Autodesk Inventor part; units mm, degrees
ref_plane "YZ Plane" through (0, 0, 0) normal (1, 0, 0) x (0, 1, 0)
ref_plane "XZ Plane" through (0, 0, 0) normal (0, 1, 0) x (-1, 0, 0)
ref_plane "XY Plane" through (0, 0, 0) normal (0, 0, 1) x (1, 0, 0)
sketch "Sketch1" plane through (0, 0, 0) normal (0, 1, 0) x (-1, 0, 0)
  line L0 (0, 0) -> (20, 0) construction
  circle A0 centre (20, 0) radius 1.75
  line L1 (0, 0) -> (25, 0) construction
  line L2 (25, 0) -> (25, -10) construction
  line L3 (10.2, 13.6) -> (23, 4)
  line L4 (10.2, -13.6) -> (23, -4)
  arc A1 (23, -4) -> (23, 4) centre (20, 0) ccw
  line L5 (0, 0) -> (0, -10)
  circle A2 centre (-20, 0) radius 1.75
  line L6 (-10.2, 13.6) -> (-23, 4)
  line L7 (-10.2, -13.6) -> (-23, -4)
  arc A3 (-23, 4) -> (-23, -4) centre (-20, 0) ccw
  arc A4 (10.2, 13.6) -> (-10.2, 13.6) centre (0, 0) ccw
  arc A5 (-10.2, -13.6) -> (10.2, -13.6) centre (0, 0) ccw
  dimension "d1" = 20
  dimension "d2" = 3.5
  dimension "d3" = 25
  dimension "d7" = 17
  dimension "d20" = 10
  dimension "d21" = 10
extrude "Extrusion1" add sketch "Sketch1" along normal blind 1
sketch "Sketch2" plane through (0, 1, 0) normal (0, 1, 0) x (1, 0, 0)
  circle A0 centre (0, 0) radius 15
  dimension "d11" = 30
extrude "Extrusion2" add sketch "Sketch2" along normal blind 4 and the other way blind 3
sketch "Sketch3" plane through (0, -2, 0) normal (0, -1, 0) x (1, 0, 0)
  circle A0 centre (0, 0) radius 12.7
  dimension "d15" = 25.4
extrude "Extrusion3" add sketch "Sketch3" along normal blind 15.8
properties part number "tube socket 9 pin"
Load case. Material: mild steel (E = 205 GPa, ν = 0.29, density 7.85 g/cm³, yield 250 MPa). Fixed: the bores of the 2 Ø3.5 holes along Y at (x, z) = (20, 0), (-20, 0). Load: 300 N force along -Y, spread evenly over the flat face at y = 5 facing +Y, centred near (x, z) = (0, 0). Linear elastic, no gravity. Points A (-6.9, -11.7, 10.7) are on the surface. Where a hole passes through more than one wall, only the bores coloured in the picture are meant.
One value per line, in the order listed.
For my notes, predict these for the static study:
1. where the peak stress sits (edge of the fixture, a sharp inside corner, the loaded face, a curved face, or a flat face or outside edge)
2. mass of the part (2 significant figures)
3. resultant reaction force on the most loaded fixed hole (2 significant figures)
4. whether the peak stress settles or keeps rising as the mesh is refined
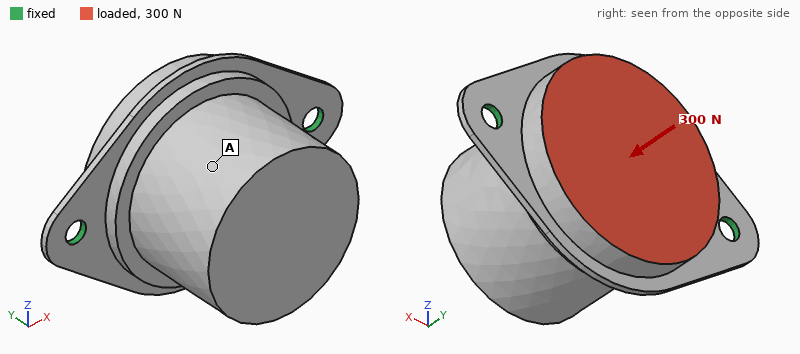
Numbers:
edge of the fixture
100 g
150 N
keeps rising
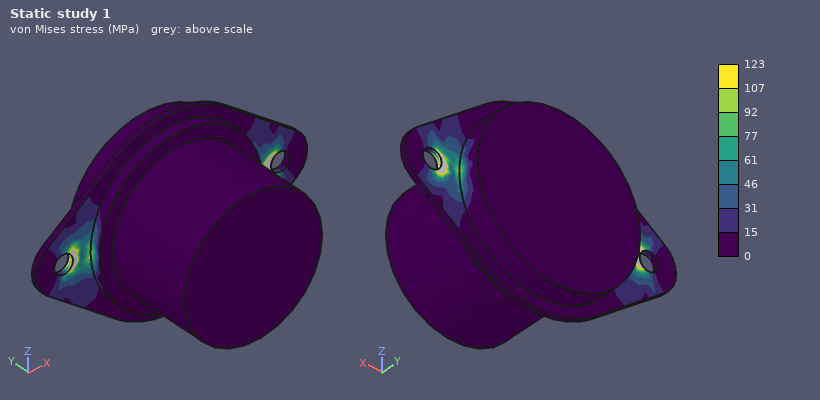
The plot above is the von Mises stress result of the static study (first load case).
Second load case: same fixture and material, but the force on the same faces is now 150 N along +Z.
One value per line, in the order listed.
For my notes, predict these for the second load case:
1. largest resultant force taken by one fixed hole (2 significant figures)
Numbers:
75 N
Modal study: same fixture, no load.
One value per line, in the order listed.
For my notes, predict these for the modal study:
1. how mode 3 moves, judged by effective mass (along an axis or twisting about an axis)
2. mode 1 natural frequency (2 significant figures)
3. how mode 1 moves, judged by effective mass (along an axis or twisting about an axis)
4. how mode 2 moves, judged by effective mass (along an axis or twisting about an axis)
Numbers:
along X
780 Hz
along Z
along Y
